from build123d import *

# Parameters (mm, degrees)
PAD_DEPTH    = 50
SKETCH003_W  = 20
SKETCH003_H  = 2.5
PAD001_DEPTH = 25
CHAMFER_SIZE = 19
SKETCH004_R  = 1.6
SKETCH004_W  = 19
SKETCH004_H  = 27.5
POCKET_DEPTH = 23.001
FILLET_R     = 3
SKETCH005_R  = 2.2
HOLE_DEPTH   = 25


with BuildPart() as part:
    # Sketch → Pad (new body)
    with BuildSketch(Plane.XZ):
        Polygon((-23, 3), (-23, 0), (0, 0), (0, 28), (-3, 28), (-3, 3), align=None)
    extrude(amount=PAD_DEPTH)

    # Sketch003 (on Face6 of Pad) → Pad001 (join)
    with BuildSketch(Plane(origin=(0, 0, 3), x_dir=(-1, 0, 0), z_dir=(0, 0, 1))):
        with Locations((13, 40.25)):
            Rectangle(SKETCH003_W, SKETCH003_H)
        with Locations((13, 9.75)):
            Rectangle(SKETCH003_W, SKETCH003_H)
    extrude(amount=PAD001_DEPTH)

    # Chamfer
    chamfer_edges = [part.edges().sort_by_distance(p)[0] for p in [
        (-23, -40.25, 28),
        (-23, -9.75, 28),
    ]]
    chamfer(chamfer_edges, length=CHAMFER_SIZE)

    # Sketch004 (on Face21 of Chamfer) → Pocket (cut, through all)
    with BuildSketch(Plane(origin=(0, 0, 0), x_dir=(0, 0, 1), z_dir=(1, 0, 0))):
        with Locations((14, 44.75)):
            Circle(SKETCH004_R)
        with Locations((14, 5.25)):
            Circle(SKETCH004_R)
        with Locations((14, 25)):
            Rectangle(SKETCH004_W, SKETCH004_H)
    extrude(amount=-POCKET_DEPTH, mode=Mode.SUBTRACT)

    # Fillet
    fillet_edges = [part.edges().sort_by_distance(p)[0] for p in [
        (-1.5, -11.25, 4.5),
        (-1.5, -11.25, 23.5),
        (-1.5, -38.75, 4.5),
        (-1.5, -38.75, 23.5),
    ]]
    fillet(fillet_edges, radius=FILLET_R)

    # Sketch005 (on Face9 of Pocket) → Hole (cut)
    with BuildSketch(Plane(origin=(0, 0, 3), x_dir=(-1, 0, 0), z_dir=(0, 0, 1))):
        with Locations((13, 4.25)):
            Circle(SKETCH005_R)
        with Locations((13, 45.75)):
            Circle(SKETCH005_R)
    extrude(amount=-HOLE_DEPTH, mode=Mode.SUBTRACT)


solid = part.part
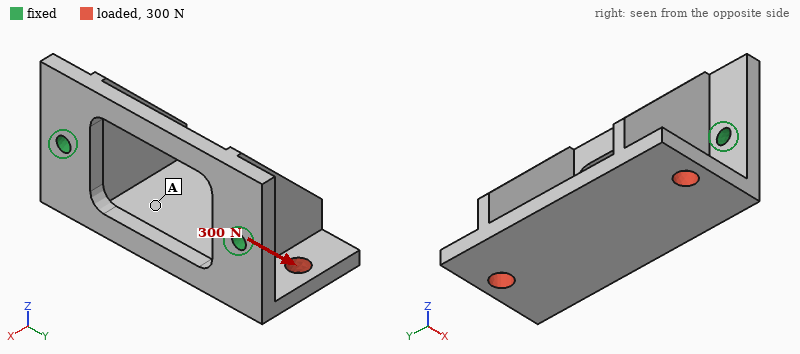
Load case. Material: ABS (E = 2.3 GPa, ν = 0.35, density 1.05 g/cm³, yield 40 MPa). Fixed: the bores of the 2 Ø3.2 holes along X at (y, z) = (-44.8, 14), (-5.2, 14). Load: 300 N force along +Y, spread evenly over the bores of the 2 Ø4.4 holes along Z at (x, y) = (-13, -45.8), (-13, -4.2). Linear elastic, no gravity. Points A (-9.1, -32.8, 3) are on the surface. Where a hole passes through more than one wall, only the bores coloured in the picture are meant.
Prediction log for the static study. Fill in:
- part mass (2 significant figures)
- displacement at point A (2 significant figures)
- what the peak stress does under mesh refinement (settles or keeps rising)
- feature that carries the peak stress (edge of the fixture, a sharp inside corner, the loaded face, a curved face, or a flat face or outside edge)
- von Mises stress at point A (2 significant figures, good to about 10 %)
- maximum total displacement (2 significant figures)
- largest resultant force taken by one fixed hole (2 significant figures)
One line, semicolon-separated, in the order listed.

7.5 g; 0.32 mm; keeps rising; edge of the fixture; 7.8 MPa; 0.61 mm; 180 N
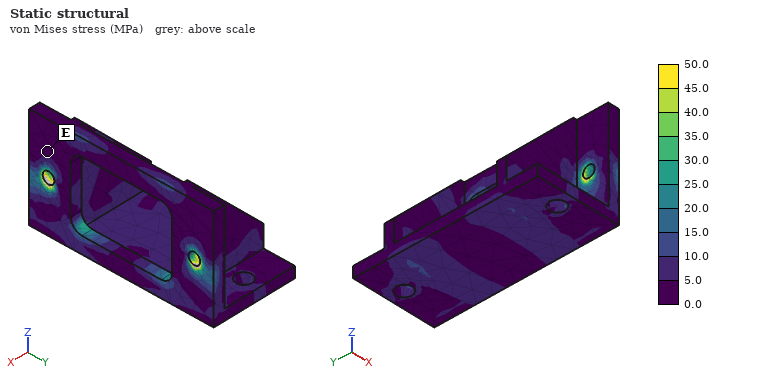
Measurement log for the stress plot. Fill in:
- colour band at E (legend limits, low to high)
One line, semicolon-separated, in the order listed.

0.0 to 5.0 MPa
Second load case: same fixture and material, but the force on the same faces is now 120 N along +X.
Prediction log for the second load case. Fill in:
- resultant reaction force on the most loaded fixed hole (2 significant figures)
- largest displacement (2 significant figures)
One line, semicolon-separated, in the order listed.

61 N; 0.52 mm
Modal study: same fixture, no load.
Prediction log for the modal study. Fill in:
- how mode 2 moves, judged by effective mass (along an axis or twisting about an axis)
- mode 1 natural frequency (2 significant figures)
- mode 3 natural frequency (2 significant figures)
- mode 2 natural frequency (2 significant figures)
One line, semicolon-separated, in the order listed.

along Y; 1100 Hz; 3000 Hz; 1600 Hz
